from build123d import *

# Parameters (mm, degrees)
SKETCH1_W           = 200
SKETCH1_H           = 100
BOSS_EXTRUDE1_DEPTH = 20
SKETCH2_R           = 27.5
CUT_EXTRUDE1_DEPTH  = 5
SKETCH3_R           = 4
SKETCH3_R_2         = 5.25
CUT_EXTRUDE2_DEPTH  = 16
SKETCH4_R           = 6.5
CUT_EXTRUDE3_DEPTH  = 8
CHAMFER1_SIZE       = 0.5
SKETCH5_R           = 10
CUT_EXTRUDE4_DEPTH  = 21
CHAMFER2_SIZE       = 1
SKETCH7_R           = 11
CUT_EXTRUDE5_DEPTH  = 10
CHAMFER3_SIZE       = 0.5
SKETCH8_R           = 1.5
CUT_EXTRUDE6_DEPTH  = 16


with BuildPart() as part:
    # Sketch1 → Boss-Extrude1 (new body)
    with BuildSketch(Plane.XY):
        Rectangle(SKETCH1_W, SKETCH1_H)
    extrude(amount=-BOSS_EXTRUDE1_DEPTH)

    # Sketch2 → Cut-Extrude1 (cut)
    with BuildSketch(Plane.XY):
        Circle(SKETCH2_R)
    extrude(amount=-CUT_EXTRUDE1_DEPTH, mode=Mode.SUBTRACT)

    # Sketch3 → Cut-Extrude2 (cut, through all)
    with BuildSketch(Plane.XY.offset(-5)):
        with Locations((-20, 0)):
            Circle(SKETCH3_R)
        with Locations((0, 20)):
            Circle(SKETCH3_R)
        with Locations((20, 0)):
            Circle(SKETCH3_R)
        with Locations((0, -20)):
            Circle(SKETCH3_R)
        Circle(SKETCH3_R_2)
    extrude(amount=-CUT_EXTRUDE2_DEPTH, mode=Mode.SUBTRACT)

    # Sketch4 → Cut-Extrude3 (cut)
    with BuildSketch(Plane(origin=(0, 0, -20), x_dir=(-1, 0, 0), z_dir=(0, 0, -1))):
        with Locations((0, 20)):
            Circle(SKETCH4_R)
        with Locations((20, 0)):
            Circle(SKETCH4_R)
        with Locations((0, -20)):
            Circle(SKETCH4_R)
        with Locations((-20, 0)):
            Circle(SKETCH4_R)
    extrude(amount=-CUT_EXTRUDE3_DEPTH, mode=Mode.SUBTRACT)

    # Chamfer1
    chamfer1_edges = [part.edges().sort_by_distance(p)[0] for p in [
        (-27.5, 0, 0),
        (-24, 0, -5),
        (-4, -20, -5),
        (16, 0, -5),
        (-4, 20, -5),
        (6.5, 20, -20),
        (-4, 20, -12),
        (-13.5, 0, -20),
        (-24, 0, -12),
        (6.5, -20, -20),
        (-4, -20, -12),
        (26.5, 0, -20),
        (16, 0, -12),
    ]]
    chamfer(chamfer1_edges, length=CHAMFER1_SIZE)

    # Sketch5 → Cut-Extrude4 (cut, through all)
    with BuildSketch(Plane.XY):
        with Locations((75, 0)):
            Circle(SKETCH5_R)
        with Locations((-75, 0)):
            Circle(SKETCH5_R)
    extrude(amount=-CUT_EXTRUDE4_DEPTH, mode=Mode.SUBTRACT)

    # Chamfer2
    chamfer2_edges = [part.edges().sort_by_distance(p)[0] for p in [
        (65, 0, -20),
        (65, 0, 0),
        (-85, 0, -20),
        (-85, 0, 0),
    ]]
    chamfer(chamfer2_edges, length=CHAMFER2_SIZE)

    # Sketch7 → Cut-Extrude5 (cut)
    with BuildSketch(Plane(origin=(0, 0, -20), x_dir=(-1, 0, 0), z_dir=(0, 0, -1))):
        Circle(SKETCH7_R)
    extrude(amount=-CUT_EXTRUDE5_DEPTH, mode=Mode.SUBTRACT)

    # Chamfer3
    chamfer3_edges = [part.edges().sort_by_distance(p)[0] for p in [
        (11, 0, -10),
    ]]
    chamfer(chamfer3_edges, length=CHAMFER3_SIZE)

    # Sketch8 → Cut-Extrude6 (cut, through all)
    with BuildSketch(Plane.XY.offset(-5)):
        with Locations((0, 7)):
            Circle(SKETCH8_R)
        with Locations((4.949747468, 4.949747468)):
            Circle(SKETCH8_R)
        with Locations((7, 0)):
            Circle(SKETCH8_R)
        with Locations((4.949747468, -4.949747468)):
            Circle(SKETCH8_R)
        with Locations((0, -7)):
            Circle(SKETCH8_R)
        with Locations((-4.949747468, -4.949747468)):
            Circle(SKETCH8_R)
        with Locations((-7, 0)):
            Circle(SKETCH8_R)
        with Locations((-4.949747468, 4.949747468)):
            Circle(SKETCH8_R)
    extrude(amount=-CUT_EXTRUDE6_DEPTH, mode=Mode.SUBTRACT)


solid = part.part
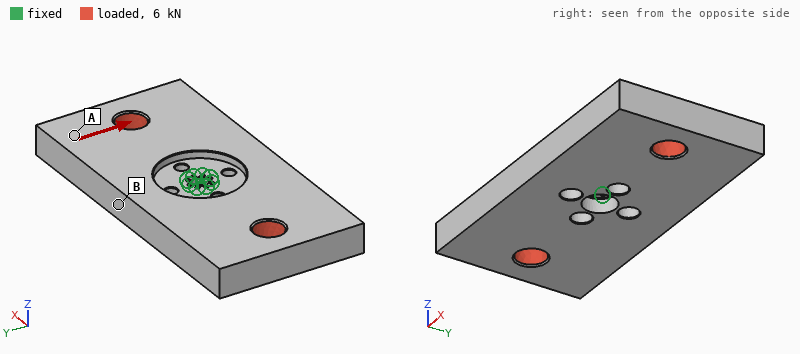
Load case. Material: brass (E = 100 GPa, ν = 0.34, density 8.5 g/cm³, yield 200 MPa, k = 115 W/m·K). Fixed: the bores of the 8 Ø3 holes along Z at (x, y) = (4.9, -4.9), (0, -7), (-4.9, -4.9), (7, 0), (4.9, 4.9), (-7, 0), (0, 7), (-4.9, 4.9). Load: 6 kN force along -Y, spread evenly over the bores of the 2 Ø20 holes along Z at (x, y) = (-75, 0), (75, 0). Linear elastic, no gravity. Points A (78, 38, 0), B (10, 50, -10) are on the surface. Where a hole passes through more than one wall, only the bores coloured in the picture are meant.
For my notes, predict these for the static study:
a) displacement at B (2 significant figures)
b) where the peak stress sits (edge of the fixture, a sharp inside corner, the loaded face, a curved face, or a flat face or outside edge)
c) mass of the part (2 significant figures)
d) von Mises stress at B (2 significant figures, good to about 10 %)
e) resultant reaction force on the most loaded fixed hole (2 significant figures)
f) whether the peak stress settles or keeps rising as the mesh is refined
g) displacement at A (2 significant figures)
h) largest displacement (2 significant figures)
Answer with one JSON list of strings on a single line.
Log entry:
["17 µm", "edge of the fixture", "3.1 kg", "7.5 MPa", "1000 N", "keeps rising", "14 µm", "23 µm"]
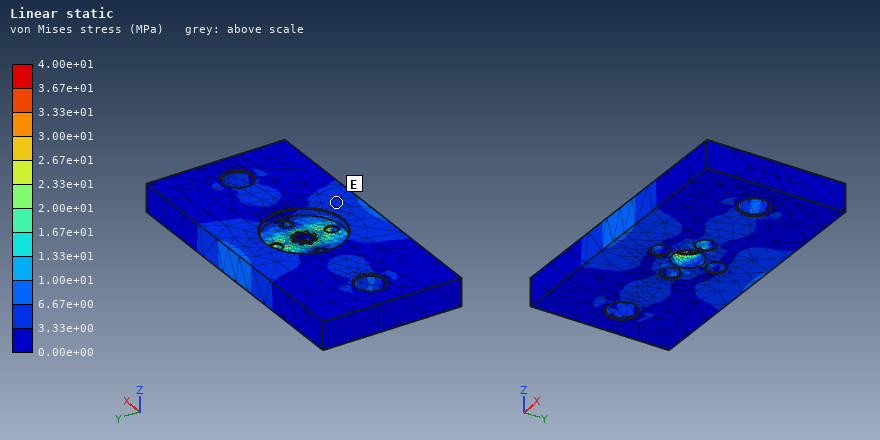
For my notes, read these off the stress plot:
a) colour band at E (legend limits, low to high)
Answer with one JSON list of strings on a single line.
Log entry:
["3.33e+00 to 6.67e+00 MPa"]
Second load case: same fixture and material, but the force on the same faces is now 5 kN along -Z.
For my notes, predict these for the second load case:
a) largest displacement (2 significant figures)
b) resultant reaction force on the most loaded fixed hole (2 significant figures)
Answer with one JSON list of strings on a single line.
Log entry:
["0.13 mm", "1.1 kN"]
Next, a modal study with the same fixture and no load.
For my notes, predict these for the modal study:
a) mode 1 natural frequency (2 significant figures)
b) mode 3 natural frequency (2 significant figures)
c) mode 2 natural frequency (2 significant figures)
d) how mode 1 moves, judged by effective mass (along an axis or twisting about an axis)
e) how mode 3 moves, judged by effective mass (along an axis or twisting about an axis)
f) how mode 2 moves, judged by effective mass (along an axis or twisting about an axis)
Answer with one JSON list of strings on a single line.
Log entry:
["330 Hz", "630 Hz", "590 Hz", "twisting about Y", "twisting about X", "twisting about Z"]
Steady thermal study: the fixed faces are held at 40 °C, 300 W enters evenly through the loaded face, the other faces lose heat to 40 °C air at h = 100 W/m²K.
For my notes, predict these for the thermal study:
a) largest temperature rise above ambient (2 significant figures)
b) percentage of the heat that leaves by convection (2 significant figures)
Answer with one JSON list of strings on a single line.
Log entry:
["60 K", "65 %"]
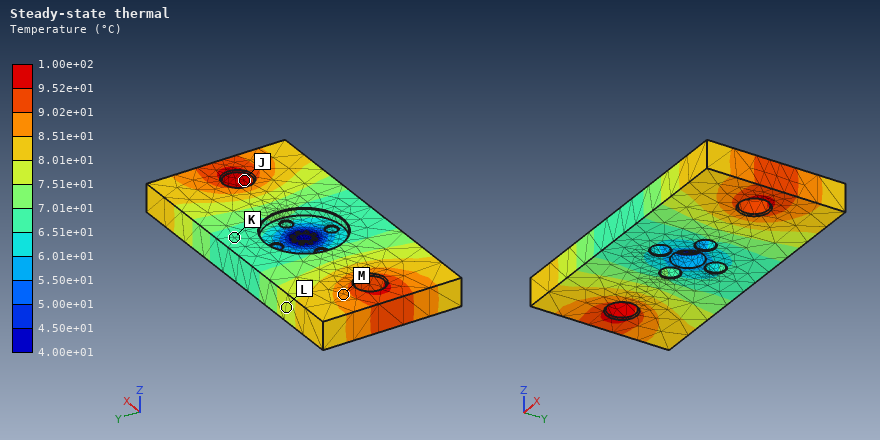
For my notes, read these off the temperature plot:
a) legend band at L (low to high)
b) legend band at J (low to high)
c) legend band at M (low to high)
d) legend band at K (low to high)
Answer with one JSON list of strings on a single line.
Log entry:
["7.51e+01 to 8.01e+01 °C", "9.52e+01 to 1.00e+02 °C", "8.51e+01 to 9.02e+01 °C", "6.51e+01 to 7.01e+01 °C"]
